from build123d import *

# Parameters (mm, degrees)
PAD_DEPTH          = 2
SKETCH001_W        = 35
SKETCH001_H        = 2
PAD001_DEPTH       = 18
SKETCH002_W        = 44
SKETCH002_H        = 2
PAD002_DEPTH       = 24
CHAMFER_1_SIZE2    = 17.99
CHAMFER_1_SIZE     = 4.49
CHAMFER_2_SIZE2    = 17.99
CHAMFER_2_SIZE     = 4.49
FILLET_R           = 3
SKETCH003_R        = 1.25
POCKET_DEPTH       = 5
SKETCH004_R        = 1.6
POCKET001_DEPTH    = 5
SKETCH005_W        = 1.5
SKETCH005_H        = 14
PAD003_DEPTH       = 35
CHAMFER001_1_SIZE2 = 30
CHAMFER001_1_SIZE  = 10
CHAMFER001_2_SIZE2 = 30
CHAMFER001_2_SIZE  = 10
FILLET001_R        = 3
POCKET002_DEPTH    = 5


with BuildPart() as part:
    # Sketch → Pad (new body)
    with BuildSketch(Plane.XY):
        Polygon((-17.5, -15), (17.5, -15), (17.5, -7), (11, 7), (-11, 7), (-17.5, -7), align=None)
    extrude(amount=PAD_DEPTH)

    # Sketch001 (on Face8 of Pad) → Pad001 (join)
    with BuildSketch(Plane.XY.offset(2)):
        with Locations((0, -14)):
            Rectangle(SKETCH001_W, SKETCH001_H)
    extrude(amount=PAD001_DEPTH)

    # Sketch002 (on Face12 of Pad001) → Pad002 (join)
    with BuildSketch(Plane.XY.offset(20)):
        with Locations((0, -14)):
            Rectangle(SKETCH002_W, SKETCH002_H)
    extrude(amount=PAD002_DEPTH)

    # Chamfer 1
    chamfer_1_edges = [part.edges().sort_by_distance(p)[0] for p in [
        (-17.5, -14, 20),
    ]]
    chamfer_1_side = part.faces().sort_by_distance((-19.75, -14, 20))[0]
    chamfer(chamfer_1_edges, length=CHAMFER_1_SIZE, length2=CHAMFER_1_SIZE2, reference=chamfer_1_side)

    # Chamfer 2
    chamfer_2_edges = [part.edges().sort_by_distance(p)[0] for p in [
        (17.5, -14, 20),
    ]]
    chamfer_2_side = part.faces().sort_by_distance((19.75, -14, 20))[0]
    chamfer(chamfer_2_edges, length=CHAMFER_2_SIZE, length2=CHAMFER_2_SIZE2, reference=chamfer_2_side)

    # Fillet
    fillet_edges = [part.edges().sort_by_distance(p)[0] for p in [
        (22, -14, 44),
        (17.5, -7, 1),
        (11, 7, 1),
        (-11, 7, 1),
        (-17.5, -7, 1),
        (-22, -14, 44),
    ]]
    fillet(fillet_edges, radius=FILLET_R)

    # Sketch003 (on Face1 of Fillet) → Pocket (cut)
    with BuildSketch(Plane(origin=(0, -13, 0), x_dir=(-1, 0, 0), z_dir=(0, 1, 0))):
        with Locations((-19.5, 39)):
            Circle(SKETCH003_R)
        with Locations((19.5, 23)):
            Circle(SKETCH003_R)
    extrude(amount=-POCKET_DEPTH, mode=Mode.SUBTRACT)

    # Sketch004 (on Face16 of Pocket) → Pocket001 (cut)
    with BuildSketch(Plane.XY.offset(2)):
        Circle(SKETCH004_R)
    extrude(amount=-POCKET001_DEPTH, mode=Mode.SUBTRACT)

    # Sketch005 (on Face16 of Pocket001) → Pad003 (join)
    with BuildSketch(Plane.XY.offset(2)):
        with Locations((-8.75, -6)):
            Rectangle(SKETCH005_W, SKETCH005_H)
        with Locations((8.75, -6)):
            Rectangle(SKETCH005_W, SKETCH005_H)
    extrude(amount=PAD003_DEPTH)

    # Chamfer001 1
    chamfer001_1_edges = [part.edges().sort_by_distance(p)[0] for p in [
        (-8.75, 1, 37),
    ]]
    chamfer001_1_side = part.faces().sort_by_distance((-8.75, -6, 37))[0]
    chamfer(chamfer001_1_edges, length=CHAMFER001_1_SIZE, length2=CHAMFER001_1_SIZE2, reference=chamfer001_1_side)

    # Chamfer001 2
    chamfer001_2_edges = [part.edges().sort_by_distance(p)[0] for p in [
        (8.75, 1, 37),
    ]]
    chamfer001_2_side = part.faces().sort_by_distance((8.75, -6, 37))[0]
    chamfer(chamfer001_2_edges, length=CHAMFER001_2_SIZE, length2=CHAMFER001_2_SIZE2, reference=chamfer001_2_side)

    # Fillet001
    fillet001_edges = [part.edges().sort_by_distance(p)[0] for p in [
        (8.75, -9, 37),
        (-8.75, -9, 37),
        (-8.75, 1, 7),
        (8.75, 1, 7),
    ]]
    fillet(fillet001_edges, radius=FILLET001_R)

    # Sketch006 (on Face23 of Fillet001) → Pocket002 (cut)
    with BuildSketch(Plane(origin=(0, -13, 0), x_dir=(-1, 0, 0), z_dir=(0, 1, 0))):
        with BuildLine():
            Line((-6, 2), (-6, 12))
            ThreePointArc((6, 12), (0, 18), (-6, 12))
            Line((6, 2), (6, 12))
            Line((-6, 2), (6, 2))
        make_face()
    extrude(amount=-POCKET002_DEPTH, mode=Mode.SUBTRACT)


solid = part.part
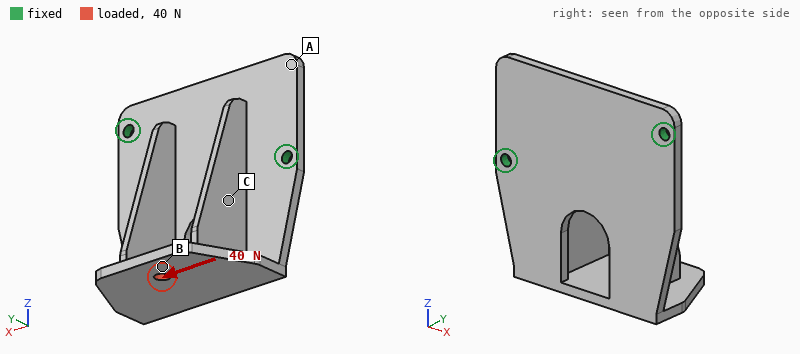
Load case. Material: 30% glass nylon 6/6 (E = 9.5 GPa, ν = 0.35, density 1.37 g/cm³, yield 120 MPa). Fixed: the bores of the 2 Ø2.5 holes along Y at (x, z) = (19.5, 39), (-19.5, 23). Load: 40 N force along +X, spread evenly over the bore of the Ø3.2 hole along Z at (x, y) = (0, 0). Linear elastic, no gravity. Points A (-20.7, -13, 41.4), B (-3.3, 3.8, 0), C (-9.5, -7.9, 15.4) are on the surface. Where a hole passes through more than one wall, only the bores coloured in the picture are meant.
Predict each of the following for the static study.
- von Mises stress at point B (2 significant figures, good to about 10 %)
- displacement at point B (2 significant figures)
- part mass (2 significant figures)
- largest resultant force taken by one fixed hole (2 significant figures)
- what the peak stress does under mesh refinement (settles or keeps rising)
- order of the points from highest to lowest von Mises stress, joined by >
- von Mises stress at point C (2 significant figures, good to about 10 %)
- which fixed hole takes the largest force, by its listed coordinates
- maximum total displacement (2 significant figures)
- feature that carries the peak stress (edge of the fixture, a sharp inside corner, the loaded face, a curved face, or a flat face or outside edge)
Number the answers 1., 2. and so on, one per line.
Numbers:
1. 4.9 MPa
2. 0.43 mm
3. 7.5 g
4. 42 N
5. keeps rising
6. C > B > A
7. 8.6 MPa
8. (-19.5, 23)
9. 0.69 mm
10. edge of the fixture
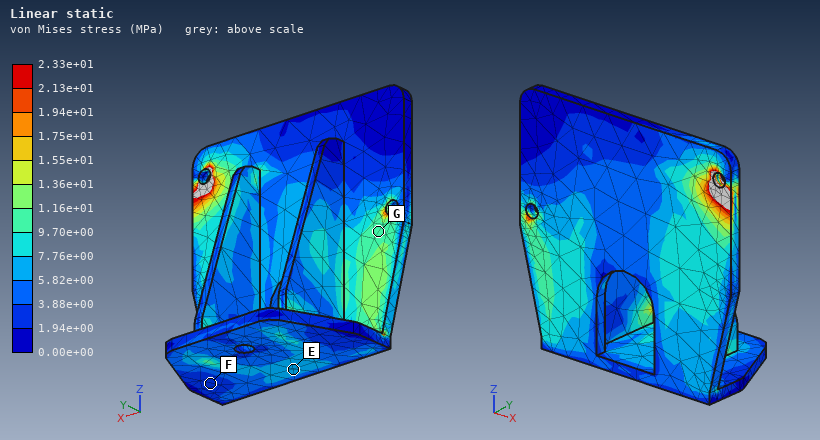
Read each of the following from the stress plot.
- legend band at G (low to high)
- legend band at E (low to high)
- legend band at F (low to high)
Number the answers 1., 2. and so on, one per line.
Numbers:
1. 9.70e+00 to 1.16e+01 MPa
2. 5.82e+00 to 7.76e+00 MPa
3. 1.94e+00 to 3.88e+00 MPa
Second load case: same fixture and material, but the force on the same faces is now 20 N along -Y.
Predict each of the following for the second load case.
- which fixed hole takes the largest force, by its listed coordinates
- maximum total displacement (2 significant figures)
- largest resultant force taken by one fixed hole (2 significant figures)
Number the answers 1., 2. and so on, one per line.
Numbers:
1. (-19.5, 23)
2. 0.72 mm
3. 16 N
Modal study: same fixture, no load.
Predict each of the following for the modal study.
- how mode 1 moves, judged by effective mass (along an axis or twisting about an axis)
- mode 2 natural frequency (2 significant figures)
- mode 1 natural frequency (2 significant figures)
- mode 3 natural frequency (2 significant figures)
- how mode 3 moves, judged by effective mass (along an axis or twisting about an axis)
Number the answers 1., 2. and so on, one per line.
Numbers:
1. along Y
2. 1400 Hz
3. 530 Hz
4. 2400 Hz
5. along Y
